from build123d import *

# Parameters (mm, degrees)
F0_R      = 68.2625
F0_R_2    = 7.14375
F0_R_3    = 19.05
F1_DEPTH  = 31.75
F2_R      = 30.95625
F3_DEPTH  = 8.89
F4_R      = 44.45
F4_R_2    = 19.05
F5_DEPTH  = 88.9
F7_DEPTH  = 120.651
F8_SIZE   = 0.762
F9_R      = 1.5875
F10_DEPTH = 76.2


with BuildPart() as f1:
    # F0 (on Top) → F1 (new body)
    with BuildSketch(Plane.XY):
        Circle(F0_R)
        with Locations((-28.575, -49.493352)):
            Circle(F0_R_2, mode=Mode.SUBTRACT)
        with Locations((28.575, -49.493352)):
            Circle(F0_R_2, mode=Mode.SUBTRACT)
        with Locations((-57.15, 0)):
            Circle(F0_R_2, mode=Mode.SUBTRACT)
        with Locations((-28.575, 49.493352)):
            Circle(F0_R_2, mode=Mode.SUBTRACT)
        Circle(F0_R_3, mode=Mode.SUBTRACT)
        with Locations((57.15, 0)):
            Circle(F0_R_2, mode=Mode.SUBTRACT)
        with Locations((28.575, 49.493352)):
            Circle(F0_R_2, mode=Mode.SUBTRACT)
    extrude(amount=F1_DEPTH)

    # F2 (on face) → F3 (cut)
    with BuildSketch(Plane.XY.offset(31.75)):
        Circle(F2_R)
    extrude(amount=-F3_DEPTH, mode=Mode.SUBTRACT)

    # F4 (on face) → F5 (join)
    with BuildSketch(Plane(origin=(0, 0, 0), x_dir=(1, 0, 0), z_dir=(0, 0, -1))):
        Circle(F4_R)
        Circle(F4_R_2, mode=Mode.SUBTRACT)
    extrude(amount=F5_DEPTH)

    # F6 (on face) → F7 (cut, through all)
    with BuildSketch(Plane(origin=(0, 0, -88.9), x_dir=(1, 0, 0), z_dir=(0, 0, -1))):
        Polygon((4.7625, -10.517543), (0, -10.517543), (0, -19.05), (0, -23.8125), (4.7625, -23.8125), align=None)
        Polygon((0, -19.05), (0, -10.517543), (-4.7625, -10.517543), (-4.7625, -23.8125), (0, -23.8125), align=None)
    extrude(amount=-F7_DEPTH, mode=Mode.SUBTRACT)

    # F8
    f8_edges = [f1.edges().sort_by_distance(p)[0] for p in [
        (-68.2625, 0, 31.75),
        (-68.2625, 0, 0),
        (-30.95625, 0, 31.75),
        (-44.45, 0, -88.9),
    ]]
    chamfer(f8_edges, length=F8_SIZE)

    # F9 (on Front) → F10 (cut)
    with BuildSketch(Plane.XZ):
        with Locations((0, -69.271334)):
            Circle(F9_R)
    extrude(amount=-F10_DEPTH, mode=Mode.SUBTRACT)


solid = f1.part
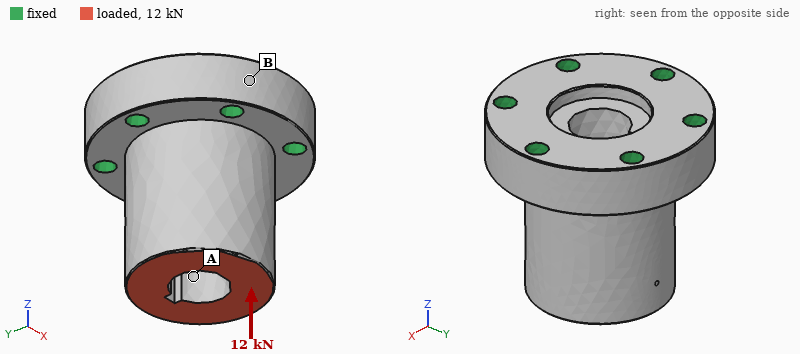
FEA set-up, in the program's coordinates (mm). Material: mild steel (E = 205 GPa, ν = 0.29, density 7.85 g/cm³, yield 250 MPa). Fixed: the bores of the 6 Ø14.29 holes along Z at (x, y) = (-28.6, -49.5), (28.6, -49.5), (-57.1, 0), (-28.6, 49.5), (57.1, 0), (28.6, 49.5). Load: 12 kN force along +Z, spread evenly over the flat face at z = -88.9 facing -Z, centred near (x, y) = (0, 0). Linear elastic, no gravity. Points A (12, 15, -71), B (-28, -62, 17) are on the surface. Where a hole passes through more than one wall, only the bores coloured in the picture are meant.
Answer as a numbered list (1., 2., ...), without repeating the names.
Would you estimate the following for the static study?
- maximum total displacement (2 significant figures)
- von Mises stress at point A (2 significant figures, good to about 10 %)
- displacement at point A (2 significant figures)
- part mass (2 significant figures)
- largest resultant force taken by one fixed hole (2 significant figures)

1. 1.5 µm
2. 2.6 MPa
3. 1.3 µm
4. 6.5 kg
5. 2.2 kN
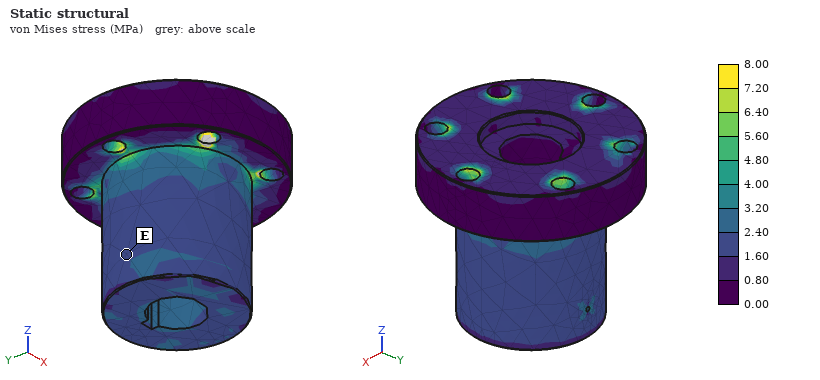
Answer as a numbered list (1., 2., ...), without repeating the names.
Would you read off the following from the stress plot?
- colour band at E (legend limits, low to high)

1. 1.60 to 2.40 MPa
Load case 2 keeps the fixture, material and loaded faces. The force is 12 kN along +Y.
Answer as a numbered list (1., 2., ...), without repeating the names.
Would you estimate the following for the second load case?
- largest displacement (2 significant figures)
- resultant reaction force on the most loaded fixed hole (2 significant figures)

1. 15 µm
2. 7.4 kN
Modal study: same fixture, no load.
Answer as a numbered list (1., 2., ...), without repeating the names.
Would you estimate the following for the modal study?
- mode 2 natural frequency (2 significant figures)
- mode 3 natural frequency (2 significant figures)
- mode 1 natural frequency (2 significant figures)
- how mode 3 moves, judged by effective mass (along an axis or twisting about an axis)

1. 4400 Hz
2. 8000 Hz
3. 4300 Hz
4. twisting about Z
